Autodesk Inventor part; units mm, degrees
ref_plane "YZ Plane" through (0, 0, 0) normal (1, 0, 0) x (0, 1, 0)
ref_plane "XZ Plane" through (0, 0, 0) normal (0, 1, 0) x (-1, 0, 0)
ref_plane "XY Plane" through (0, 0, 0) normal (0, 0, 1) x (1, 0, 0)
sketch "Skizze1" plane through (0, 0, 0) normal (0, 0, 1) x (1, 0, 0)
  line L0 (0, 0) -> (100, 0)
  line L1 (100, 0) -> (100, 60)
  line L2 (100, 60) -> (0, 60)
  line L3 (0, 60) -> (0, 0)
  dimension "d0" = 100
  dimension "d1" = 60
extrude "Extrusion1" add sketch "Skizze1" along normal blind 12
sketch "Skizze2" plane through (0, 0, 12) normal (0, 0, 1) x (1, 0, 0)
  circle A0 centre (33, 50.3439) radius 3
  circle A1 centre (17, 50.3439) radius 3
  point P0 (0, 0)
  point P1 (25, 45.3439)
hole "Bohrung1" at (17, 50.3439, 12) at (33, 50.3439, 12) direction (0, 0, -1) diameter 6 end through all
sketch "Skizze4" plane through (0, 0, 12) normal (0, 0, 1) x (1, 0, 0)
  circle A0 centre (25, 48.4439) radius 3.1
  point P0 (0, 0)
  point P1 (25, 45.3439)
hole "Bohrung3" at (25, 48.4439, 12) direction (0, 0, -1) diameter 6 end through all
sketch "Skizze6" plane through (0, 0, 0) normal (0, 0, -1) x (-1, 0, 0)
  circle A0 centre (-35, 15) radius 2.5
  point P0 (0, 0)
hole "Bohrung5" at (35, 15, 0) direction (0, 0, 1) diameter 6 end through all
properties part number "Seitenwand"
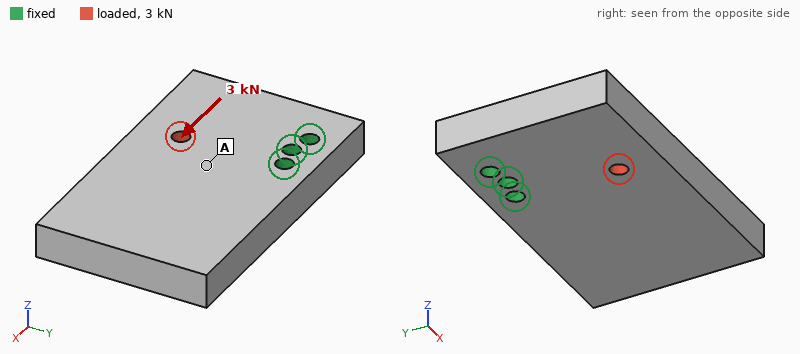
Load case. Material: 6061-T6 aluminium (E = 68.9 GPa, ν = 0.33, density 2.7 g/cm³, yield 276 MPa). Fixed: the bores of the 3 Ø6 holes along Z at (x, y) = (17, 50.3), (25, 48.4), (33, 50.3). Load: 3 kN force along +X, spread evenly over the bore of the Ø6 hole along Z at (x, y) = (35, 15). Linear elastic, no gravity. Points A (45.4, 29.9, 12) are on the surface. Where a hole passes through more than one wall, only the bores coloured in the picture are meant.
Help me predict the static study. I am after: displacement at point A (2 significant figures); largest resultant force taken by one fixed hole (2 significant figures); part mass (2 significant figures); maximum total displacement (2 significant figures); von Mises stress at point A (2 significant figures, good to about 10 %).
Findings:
17 µm
4.4 kN
190 g
56 µm
6.7 MPa
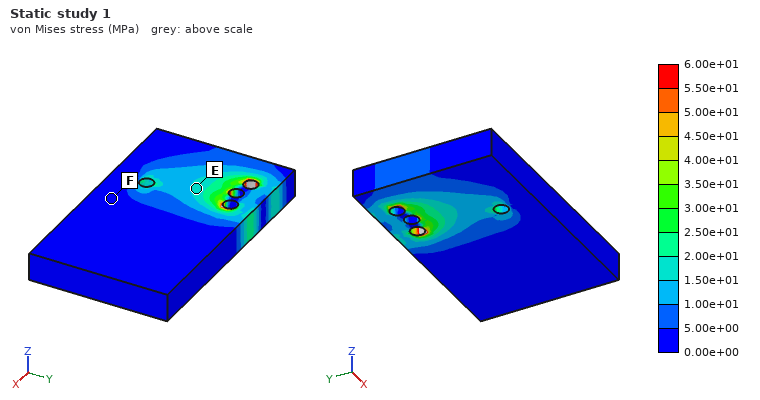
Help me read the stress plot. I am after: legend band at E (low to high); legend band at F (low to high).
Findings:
1.50e+01 to 2.00e+01 MPa
0.00e+00 to 5.00e+00 MPa
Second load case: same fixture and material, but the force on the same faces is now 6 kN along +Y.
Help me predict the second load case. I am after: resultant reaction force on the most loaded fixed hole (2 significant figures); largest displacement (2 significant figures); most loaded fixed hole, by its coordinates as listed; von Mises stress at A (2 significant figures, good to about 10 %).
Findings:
5.0 kN
30 µm
(33, 50.3)
12 MPa
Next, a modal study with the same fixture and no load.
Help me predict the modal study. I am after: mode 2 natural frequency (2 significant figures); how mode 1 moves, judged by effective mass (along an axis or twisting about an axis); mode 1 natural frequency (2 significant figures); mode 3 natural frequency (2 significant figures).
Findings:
3100 Hz
along Z
1600 Hz
3200 Hz
